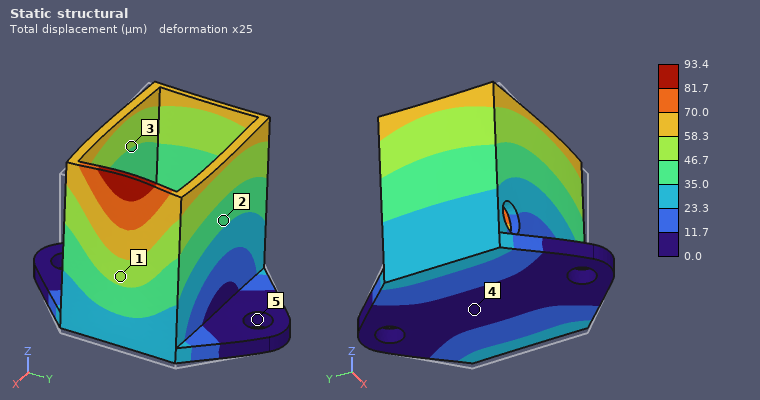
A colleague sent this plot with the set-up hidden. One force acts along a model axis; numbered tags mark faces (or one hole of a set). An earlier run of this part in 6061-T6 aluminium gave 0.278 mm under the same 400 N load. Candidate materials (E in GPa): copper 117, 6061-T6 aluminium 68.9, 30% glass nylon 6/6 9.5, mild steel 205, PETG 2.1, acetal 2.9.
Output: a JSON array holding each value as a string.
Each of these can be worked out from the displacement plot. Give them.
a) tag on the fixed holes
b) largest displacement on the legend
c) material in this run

["5", "93.4 µm", "mild steel"]
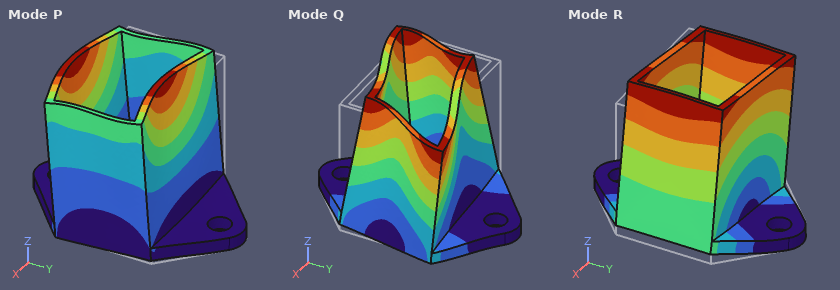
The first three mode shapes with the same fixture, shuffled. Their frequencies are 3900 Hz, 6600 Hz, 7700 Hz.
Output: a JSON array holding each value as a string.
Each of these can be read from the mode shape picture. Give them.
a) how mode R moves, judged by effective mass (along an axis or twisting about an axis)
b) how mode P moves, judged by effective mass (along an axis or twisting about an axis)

["along X", "along Y"]
